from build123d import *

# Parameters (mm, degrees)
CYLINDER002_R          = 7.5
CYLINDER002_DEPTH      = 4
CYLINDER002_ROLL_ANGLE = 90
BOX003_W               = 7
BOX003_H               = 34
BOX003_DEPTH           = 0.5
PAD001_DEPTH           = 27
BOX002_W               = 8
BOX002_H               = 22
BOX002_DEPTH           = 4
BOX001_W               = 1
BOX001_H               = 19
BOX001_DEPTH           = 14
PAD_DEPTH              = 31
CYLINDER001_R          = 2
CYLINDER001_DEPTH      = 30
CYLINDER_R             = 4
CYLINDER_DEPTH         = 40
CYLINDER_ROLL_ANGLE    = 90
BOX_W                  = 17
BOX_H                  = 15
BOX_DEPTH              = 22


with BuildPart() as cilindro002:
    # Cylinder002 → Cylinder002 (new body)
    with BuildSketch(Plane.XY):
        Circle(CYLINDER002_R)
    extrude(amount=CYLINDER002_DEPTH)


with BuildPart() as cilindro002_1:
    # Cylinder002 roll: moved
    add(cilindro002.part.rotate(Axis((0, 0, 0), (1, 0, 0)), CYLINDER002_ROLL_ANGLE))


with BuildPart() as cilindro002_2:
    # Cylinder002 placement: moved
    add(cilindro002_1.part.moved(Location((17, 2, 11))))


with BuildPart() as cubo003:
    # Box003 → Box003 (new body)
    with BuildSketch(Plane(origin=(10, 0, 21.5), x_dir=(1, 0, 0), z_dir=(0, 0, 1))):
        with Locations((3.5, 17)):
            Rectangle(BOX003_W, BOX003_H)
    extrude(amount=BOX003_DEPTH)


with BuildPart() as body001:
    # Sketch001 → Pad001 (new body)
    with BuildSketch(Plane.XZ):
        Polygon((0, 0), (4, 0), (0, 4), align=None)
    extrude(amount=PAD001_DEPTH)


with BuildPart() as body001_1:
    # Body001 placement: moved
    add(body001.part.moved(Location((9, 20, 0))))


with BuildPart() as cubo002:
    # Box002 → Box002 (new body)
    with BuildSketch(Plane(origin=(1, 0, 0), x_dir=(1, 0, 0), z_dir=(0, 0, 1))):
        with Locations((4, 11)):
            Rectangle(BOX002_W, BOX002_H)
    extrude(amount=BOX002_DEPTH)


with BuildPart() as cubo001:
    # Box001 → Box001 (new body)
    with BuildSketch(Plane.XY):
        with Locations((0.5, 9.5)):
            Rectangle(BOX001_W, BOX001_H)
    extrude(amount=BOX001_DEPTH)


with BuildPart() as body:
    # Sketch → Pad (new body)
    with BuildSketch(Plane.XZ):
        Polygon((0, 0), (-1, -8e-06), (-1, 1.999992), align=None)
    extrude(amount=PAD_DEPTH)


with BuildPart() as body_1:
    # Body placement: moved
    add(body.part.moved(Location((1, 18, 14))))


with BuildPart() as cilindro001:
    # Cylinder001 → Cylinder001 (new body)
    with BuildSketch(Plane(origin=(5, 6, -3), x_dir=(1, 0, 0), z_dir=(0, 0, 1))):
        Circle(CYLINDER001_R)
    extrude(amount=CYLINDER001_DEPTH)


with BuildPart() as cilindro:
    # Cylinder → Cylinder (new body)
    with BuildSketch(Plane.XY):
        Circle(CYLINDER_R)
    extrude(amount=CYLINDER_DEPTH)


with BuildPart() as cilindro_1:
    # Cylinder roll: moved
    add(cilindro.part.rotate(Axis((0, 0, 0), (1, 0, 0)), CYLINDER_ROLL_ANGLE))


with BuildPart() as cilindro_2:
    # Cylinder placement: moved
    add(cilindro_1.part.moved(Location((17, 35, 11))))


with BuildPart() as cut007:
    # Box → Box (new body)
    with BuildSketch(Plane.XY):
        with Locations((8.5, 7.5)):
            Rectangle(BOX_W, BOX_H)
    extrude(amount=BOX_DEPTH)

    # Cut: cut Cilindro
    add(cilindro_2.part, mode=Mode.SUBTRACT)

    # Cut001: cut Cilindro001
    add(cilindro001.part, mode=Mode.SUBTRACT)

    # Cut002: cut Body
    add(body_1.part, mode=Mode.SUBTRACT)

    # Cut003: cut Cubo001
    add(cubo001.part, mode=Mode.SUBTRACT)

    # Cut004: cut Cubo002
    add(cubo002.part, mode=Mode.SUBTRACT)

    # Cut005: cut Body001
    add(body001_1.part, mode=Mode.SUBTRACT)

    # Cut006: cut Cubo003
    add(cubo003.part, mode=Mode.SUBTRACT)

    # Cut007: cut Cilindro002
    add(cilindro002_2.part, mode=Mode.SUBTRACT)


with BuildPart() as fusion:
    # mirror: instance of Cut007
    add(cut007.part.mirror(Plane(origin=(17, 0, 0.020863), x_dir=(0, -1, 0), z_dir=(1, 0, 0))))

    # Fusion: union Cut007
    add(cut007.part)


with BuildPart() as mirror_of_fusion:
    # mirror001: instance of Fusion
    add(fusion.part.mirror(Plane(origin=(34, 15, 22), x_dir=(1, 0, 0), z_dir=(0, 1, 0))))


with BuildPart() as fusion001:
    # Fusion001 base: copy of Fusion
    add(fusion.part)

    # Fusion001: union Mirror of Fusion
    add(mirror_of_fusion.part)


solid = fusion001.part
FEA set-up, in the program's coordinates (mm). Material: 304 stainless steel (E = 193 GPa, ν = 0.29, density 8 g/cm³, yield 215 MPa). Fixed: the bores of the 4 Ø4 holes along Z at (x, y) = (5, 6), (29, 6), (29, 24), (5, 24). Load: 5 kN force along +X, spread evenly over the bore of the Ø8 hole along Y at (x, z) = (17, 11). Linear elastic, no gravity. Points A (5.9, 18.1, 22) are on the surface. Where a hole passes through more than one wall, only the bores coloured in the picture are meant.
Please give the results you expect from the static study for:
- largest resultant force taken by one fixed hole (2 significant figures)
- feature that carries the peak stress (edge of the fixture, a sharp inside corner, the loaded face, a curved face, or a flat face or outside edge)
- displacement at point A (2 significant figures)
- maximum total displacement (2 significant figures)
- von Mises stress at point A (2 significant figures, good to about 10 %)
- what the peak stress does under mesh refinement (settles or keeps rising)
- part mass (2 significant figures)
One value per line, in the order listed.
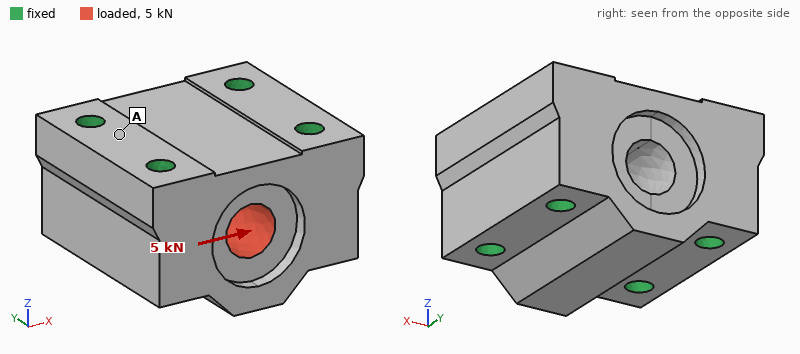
2.0 kN
edge of the fixture
0.13 µm
0.80 µm
2.9 MPa
keeps rising
130 g
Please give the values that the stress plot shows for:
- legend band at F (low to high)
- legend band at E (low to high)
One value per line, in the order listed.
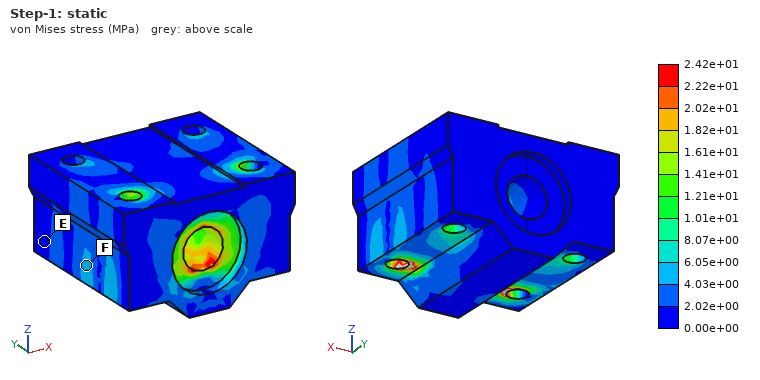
4.03e+00 to 6.05e+00 MPa
0.00e+00 to 2.02e+00 MPa
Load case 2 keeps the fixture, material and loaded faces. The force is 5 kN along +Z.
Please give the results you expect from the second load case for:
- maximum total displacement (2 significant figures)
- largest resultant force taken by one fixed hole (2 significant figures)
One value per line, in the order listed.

1.6 µm
2.0 kN
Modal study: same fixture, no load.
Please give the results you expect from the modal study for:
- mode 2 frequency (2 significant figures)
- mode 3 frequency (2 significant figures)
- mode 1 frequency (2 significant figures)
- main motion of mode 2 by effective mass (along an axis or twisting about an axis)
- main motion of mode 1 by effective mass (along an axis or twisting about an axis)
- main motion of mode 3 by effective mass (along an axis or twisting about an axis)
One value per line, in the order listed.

56 kHz
64 kHz
52 kHz
along Z
along Y
along Y
